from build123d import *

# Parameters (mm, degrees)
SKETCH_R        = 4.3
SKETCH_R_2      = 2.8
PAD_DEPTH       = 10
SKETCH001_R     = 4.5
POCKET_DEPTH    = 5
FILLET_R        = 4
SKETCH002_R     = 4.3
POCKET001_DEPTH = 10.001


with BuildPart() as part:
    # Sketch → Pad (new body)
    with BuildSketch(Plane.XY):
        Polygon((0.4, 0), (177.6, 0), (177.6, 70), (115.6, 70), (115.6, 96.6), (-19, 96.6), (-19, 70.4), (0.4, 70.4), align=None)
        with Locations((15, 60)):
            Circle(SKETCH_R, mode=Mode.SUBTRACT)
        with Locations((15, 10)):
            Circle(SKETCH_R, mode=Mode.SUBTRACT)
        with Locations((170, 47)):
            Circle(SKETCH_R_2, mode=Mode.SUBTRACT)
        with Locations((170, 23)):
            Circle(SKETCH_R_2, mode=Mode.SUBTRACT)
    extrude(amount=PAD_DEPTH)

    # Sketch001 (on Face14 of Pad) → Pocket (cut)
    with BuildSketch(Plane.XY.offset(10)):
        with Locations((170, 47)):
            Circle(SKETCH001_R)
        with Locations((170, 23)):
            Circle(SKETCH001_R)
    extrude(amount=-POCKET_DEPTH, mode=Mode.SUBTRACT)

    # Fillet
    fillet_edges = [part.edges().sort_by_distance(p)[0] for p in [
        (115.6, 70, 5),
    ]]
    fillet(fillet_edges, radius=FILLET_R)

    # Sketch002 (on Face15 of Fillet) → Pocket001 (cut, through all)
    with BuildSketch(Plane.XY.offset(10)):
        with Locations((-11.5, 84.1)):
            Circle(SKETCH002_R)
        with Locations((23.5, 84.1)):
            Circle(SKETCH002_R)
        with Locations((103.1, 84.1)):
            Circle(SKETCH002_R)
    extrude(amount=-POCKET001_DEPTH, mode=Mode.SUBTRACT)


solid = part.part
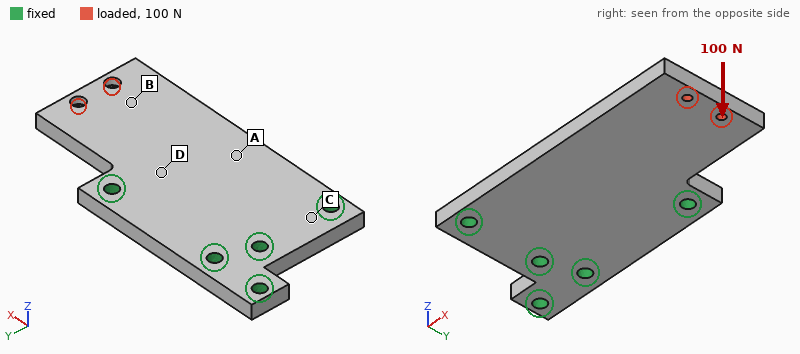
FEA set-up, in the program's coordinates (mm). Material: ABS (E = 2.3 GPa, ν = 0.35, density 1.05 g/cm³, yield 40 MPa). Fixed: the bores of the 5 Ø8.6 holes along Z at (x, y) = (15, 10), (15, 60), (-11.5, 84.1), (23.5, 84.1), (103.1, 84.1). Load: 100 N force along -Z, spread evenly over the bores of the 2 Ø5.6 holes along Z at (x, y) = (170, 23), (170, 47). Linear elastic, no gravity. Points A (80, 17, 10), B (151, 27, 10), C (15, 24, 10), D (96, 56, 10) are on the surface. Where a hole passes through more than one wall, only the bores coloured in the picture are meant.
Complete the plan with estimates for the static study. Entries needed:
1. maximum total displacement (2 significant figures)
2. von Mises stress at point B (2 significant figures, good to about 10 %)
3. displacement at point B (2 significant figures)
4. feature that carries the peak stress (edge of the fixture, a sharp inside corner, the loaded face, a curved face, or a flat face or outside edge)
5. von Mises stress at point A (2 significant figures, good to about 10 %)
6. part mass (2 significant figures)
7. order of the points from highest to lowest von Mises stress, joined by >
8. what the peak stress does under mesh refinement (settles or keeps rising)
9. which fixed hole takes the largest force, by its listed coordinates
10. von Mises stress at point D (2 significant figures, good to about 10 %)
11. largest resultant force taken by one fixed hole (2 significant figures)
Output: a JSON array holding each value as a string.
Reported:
["2.4 mm", "2.0 MPa", "1.4 mm", "edge of the fixture", "3.0 MPa", "160 g", "D > A > B > C", "keeps rising", "(103.1, 84.1)", "4.7 MPa", "150 N"]
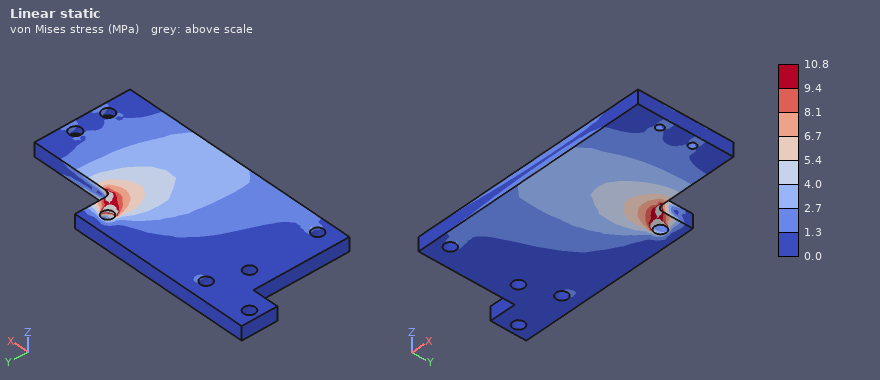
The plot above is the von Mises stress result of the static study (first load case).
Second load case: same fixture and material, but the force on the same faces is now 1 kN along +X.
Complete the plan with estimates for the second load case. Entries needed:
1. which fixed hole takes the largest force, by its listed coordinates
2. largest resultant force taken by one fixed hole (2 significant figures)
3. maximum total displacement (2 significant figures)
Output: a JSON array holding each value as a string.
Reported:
["(15, 10)", "390 N", "0.86 mm"]
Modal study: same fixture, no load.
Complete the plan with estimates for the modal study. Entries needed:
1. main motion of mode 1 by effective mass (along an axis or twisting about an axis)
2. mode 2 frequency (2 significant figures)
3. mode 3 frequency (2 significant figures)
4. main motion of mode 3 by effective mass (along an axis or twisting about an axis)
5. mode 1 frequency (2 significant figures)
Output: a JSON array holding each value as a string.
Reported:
["along Z", "570 Hz", "1000 Hz", "along Z", "230 Hz"]
